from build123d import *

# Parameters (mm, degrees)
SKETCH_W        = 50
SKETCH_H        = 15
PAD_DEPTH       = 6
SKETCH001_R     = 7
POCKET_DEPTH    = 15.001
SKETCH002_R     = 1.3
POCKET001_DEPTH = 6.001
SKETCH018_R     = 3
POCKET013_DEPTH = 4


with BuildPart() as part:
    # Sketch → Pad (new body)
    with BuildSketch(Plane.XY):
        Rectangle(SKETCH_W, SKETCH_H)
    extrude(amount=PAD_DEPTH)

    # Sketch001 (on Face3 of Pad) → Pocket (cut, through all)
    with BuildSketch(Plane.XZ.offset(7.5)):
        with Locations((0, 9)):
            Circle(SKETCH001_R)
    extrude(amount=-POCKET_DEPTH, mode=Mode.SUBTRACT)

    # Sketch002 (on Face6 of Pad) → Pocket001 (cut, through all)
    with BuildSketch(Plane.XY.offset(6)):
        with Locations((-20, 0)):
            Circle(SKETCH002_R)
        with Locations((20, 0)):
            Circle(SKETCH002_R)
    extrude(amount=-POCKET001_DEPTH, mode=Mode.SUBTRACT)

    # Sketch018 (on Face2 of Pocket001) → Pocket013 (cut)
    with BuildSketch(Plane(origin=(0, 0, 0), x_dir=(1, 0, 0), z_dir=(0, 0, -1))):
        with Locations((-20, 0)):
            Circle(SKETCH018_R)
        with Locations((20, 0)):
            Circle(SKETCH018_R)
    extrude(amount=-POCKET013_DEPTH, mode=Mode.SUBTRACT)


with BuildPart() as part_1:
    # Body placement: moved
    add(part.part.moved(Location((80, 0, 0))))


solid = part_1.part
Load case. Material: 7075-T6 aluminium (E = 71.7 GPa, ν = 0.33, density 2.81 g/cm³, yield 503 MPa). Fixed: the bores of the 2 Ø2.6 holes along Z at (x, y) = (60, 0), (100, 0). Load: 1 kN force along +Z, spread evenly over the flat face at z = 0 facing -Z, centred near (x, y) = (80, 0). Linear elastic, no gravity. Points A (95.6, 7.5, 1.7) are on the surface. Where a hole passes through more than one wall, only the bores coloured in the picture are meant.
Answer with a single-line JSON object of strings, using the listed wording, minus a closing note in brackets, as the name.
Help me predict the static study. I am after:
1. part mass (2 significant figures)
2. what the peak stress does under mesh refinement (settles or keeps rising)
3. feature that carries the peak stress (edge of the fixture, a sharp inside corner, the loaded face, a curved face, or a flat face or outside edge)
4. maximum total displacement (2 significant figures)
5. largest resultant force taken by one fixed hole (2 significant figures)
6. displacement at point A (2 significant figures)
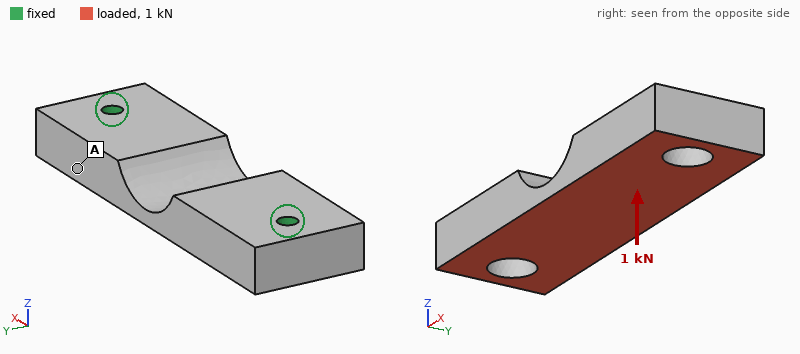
{"part mass": "10 g", "what the peak stress does under mesh refinement": "keeps rising", "feature that carries the peak stress": "edge of the fixture", "maximum total displacement": "28 µm", "largest resultant force taken by one fixed hole": "880 N", "displacement at point A": "9.3 µm"}
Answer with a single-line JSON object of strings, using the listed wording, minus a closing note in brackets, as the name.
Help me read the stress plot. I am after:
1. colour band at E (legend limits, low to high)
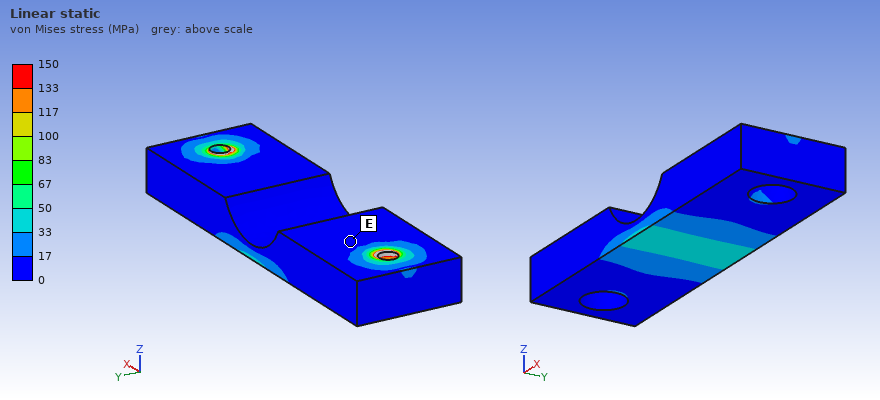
{"colour band at E": "0 to 17 MPa"}
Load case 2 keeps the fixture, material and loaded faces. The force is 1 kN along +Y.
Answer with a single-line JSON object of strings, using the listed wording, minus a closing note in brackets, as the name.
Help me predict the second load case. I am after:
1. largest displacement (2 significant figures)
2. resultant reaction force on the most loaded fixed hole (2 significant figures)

{"largest displacement": "52 µm", "resultant reaction force on the most loaded fixed hole": "500 N"}
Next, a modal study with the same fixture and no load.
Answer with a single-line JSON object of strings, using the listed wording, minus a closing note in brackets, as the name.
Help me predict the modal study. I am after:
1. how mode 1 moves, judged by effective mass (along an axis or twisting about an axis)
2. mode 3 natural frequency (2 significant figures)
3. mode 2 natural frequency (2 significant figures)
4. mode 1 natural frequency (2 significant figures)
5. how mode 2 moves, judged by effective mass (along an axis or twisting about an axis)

{"how mode 1 moves, judged by effective mass": "along Y", "mode 3 natural frequency": "17 kHz", "mode 2 natural frequency": "12 kHz", "mode 1 natural frequency": "10 kHz", "how mode 2 moves, judged by effective mass": "along Z"}
